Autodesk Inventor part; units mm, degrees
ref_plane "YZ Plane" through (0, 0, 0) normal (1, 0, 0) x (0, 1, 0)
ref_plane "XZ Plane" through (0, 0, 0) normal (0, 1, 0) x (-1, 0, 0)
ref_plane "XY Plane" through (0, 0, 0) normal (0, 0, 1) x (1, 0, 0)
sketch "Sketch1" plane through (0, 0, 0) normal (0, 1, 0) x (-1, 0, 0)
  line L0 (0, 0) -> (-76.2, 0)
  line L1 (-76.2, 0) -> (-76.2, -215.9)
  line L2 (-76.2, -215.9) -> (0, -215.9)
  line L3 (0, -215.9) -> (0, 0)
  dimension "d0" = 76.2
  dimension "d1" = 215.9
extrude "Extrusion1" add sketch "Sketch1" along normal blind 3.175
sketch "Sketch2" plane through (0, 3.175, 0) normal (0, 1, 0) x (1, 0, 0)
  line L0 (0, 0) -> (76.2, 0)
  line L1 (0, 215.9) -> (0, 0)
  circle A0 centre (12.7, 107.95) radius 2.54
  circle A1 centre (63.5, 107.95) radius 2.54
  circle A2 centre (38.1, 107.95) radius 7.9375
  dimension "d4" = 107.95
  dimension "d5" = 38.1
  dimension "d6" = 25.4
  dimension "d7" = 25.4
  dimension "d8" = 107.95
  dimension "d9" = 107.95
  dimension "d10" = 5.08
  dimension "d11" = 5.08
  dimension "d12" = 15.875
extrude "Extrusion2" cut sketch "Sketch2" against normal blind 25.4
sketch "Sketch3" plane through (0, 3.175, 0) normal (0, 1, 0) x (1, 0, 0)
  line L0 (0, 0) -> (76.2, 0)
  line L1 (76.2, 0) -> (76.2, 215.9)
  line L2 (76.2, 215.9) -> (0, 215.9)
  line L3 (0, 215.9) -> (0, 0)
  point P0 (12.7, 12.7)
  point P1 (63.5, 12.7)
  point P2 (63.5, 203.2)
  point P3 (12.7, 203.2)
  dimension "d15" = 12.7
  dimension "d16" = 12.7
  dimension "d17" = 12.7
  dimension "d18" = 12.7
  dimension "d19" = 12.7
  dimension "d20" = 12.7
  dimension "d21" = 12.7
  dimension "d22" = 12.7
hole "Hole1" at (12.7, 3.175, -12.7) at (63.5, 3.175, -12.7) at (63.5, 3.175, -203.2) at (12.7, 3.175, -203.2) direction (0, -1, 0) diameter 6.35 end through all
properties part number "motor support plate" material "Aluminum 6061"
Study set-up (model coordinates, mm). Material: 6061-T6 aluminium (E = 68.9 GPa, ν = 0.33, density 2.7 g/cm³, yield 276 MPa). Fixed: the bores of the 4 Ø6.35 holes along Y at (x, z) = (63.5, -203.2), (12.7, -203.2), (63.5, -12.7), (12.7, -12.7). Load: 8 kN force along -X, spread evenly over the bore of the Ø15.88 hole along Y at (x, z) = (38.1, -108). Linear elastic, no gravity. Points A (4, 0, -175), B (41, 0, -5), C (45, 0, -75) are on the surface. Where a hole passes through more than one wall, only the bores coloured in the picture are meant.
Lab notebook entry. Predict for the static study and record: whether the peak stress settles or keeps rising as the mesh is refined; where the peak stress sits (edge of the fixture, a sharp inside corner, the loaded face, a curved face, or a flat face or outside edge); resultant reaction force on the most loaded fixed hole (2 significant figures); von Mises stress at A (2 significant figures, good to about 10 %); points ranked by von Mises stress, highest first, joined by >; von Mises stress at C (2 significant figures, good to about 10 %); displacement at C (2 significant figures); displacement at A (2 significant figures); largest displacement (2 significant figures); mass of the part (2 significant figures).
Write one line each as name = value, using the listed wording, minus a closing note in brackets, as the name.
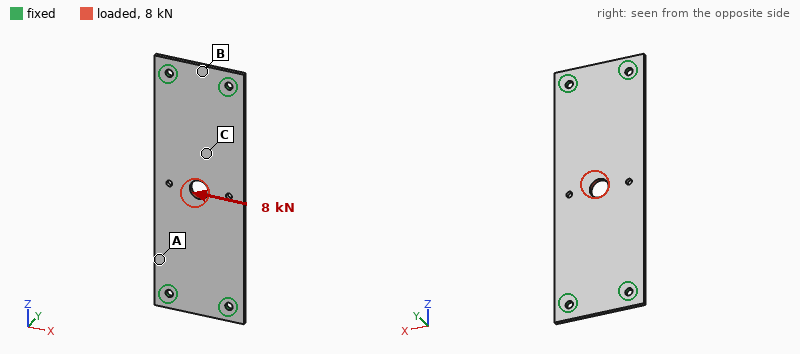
whether the peak stress settles or keeps rising as the mesh is refined = keeps rising
where the peak stress sits = edge of the fixture
resultant reaction force on the most loaded fixed hole = 3.9 kN
von Mises stress at A = 20 MPa
points ranked by von Mises stress, highest first, joined by > = C > A > B
von Mises stress at C = 39 MPa
displacement at C = 0.081 mm
displacement at A = 0.041 mm
largest displacement = 0.12 mm
mass of the part = 140 g
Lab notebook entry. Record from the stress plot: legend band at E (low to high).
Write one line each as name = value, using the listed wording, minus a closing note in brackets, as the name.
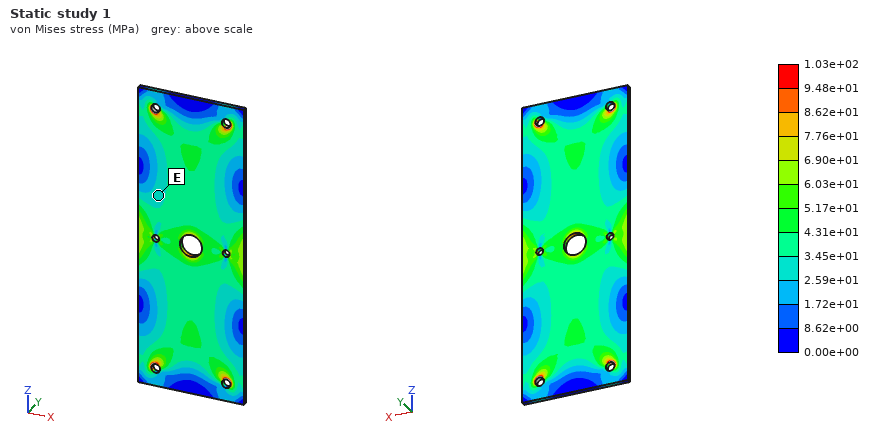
legend band at E = 2.59e+01 to 3.45e+01 MPa
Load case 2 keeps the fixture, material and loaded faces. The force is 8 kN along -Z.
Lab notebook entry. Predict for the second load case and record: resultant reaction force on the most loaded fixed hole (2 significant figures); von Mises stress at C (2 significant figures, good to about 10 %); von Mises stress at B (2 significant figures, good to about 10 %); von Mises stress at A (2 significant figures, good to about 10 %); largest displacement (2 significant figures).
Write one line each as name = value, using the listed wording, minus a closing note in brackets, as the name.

resultant reaction force on the most loaded fixed hole = 2.0 kN
von Mises stress at C = 26 MPa
von Mises stress at B = 5.8 MPa
von Mises stress at A = 18 MPa
largest displacement = 34 µm
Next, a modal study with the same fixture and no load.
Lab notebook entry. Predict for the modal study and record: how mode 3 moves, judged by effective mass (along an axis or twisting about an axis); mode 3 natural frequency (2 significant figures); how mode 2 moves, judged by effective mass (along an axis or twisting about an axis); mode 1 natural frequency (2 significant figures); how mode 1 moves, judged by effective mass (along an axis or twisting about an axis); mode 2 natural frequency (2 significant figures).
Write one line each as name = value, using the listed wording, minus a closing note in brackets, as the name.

how mode 3 moves, judged by effective mass = twisting about X
mode 3 natural frequency = 1300 Hz
how mode 2 moves, judged by effective mass = twisting about Z
mode 1 natural frequency = 460 Hz
how mode 1 moves, judged by effective mass = along Y
mode 2 natural frequency = 880 Hz
